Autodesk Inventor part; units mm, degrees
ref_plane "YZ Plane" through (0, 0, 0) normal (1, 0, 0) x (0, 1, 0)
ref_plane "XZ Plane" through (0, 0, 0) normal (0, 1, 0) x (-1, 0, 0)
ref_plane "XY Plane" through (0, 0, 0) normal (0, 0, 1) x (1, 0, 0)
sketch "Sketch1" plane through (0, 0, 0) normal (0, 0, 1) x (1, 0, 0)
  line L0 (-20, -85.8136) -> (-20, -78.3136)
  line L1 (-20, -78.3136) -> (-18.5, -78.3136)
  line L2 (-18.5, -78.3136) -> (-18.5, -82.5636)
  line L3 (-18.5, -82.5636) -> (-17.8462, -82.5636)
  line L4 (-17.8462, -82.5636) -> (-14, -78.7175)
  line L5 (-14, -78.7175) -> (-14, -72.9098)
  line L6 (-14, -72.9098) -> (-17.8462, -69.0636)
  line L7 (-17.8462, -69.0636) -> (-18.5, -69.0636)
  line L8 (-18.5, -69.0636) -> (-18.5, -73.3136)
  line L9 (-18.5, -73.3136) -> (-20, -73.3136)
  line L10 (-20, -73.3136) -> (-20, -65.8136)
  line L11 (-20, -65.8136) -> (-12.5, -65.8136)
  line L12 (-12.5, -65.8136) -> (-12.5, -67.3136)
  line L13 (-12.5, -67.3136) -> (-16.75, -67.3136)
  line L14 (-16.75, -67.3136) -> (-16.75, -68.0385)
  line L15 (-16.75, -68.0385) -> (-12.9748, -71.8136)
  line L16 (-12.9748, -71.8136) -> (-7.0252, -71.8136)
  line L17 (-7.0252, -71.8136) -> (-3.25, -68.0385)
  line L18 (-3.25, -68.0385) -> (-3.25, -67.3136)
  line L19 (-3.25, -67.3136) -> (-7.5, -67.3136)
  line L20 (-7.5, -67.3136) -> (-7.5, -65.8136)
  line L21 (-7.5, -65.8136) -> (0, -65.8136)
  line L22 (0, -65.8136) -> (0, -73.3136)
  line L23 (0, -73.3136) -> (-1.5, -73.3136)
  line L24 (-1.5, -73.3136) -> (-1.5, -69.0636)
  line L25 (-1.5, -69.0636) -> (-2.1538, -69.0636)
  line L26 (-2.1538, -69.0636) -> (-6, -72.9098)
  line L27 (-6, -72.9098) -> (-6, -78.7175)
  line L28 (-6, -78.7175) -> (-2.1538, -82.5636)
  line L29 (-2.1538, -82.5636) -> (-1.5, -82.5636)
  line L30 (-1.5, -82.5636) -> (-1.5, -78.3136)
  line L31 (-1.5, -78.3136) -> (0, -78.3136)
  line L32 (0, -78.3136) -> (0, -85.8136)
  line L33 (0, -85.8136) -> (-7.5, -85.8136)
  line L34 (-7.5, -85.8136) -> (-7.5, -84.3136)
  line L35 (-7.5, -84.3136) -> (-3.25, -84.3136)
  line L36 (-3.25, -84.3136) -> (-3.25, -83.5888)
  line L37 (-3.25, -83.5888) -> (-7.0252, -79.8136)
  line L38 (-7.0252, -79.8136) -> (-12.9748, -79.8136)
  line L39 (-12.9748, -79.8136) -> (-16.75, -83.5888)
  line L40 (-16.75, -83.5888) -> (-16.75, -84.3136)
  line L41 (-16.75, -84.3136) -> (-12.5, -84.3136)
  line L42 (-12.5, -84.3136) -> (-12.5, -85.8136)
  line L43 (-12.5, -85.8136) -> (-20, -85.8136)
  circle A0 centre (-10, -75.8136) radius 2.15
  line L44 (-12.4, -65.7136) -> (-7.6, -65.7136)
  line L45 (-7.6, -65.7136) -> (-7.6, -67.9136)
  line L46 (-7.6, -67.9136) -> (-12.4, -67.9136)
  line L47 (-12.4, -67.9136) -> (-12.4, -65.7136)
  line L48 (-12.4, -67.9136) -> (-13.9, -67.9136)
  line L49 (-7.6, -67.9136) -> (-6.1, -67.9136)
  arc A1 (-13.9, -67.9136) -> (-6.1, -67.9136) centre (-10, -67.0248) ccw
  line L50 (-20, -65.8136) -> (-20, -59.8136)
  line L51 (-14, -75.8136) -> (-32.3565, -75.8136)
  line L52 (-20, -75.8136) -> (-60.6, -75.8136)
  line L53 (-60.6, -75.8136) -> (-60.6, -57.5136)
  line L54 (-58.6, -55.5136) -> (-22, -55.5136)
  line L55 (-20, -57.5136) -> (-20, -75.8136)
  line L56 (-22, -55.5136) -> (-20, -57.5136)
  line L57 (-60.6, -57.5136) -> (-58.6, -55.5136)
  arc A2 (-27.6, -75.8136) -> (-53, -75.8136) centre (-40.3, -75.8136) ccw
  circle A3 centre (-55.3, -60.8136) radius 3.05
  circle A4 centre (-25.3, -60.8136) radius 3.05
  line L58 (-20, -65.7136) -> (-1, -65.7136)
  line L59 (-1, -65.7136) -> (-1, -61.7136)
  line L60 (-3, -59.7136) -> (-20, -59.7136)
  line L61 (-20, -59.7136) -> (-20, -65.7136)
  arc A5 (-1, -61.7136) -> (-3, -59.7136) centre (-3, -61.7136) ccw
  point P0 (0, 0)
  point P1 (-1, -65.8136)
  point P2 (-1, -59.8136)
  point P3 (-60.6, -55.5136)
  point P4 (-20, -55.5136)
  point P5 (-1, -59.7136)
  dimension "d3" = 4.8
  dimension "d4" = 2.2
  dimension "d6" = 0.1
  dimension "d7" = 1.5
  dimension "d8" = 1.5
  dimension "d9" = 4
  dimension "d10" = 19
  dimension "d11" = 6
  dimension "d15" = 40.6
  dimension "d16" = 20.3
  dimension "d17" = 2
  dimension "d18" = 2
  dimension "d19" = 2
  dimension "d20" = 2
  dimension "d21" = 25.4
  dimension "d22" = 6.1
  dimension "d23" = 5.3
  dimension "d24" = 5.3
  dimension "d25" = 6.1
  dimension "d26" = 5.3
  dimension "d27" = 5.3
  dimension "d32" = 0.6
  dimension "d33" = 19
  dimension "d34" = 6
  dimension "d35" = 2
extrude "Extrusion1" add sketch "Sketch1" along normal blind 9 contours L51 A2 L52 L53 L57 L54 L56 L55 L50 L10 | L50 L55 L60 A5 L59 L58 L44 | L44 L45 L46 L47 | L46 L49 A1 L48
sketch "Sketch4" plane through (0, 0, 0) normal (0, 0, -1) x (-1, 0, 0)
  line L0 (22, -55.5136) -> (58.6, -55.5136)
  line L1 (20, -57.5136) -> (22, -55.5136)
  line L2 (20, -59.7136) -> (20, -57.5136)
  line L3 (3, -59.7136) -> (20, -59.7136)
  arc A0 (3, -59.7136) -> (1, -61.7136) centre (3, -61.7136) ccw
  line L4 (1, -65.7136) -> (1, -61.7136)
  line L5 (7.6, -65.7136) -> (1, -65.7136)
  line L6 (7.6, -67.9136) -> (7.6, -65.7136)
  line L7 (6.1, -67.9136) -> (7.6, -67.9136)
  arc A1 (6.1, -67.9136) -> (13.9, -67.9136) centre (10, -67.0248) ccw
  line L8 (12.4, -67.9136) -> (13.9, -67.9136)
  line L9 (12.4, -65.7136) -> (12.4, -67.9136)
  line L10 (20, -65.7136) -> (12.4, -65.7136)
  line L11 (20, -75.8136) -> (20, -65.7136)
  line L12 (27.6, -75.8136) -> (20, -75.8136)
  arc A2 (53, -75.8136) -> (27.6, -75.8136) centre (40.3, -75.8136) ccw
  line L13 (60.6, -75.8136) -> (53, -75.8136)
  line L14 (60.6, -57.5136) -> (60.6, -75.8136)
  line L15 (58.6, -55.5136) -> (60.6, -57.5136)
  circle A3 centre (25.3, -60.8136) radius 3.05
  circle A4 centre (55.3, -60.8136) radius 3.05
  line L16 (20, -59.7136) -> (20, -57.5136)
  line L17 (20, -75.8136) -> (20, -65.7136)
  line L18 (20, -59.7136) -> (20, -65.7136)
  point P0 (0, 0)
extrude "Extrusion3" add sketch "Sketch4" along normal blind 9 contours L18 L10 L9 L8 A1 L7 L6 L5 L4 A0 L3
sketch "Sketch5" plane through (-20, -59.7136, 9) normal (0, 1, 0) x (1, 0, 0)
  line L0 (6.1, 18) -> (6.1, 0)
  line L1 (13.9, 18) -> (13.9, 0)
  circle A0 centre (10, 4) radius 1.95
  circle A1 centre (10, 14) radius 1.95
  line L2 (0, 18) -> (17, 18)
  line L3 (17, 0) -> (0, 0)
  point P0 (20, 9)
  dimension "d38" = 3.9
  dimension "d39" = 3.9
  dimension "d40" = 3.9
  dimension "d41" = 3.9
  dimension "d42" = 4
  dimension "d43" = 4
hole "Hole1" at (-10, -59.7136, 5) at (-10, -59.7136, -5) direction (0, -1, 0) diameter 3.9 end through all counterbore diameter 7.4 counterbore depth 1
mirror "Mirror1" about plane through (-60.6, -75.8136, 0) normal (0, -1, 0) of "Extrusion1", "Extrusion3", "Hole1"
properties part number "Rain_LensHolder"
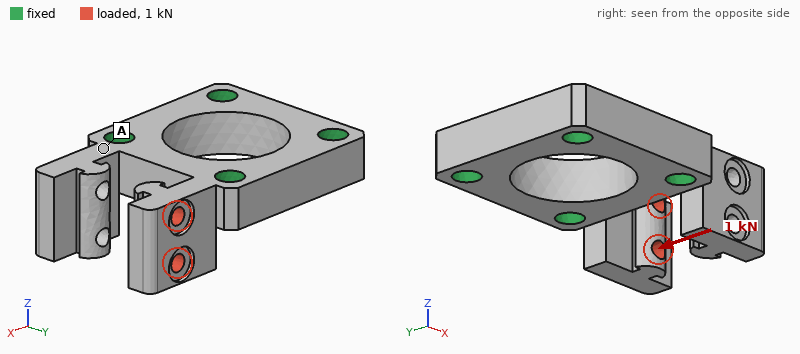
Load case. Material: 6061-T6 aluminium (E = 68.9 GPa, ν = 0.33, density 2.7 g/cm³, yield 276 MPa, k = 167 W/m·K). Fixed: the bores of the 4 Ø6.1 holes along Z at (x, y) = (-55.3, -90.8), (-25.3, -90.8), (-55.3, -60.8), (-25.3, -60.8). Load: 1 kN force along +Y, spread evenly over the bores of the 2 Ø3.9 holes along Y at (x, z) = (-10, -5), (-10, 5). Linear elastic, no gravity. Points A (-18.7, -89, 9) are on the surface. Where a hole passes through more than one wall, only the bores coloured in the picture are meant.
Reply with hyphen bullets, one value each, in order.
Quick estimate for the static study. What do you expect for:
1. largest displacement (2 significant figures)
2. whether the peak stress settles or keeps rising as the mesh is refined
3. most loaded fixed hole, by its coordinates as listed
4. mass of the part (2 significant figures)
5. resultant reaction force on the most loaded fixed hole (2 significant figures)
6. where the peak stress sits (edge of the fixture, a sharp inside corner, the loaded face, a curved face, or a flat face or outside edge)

- 0.13 mm
- keeps rising
- (-25.3, -60.8)
- 37 g
- 780 N
- a sharp inside corner
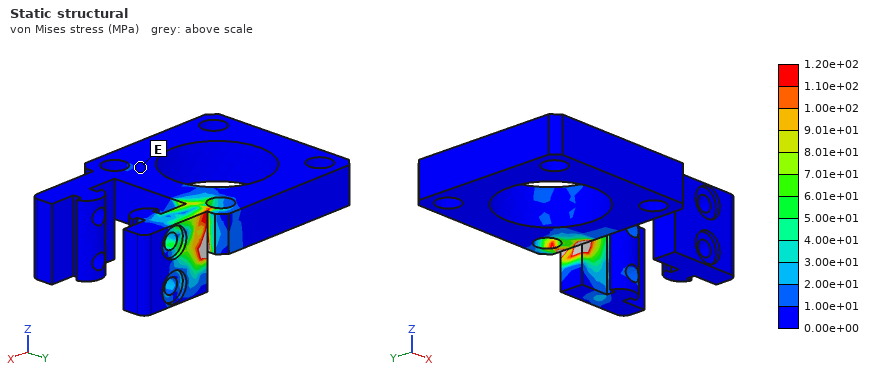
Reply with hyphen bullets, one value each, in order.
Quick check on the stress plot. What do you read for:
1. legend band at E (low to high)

- 0.00e+00 to 1.00e+01 MPa
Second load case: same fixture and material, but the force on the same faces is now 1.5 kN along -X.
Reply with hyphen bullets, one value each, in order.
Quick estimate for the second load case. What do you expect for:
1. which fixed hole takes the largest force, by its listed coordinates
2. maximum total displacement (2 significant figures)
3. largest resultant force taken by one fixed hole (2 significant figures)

- (-25.3, -60.8)
- 85 µm
- 1.4 kN
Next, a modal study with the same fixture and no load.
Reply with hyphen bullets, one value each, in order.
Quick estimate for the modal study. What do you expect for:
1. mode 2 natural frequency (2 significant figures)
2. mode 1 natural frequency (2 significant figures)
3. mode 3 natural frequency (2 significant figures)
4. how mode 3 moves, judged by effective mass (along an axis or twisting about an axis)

- 7300 Hz
- 7300 Hz
- 9300 Hz
- along Z
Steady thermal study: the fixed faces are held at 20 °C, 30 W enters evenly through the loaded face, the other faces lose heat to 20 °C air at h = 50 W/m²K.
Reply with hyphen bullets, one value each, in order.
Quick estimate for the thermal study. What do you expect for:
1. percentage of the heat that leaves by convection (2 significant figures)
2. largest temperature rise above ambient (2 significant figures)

- 6.5 %
- 37 K
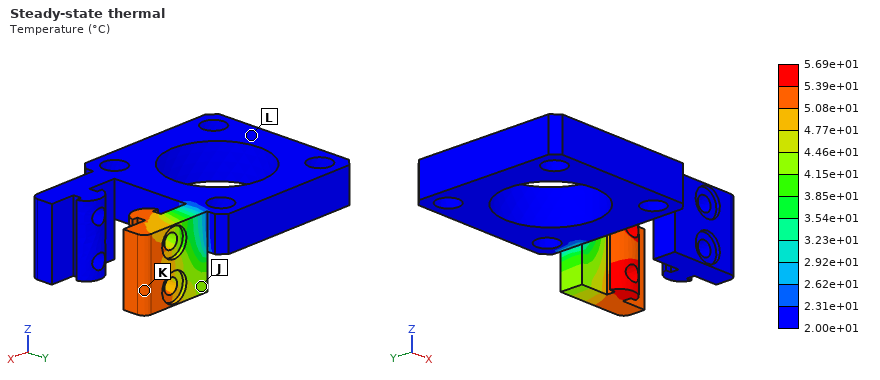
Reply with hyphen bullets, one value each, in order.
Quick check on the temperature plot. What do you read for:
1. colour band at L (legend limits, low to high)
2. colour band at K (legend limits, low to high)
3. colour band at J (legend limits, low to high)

- 2.00e+01 to 2.31e+01 °C
- 5.08e+01 to 5.39e+01 °C
- 4.15e+01 to 4.46e+01 °C
